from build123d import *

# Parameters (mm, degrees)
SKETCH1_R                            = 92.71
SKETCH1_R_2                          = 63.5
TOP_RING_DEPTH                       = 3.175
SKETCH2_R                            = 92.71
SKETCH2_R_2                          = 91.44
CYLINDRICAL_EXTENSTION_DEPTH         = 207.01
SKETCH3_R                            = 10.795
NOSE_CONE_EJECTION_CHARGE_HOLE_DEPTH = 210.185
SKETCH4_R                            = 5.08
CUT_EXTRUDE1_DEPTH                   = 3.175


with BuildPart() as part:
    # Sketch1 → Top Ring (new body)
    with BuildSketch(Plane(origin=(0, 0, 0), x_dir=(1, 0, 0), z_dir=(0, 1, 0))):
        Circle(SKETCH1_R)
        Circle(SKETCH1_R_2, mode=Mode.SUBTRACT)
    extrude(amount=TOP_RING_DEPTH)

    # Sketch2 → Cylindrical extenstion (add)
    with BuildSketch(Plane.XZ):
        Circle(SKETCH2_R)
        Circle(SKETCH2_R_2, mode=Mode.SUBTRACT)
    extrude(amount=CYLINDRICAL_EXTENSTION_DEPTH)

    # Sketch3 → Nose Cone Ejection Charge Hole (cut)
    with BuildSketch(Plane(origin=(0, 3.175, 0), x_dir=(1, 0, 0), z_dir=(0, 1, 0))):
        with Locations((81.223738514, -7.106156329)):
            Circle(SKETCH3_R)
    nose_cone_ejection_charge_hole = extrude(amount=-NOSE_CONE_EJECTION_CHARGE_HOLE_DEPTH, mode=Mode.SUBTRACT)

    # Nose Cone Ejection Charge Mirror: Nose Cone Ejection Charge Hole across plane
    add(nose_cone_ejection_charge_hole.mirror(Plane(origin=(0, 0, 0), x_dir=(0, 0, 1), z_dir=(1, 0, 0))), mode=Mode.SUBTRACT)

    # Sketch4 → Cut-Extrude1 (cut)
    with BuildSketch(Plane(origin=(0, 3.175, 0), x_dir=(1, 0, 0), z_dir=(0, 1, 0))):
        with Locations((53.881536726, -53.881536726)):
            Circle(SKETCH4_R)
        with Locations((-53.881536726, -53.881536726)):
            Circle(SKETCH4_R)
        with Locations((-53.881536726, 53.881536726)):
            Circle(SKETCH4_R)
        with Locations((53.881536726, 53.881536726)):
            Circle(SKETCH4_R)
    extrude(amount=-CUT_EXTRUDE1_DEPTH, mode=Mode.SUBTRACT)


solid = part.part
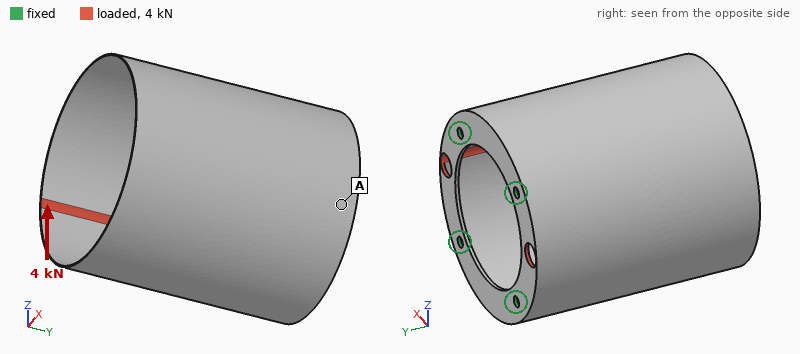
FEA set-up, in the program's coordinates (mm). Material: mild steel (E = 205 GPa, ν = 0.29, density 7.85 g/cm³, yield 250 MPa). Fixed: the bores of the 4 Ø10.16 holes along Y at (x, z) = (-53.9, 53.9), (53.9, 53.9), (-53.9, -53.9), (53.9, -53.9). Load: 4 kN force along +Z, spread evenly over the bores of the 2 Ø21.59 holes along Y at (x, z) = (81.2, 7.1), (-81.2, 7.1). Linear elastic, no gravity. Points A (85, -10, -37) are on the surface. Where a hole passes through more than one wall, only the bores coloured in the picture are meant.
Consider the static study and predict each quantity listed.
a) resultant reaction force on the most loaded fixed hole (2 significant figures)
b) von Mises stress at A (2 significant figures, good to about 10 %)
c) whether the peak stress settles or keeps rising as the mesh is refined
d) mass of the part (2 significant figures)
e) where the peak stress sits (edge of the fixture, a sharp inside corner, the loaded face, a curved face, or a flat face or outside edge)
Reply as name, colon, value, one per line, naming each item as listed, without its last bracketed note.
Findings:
resultant reaction force on the most loaded fixed hole: 1.9 kN
von Mises stress at A: 22 MPa
whether the peak stress settles or keeps rising as the mesh is refined: keeps rising
mass of the part: 1.5 kg
where the peak stress sits: edge of the fixture
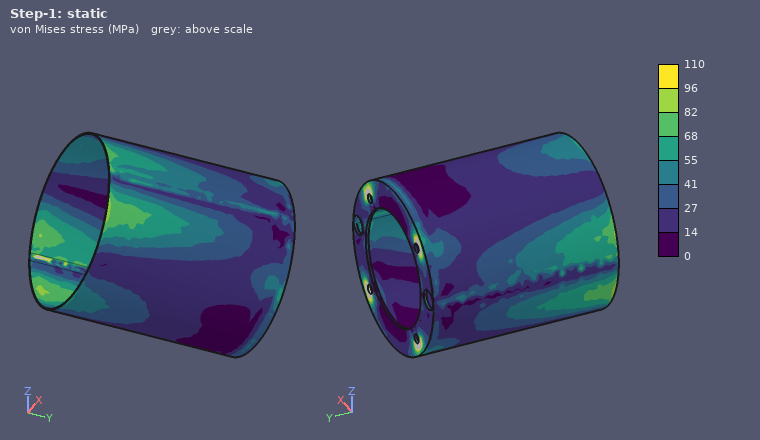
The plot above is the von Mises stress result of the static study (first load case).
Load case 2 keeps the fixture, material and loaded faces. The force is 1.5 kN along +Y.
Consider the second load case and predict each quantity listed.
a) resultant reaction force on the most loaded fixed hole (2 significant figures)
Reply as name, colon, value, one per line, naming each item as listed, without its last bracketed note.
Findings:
resultant reaction force on the most loaded fixed hole: 430 N
